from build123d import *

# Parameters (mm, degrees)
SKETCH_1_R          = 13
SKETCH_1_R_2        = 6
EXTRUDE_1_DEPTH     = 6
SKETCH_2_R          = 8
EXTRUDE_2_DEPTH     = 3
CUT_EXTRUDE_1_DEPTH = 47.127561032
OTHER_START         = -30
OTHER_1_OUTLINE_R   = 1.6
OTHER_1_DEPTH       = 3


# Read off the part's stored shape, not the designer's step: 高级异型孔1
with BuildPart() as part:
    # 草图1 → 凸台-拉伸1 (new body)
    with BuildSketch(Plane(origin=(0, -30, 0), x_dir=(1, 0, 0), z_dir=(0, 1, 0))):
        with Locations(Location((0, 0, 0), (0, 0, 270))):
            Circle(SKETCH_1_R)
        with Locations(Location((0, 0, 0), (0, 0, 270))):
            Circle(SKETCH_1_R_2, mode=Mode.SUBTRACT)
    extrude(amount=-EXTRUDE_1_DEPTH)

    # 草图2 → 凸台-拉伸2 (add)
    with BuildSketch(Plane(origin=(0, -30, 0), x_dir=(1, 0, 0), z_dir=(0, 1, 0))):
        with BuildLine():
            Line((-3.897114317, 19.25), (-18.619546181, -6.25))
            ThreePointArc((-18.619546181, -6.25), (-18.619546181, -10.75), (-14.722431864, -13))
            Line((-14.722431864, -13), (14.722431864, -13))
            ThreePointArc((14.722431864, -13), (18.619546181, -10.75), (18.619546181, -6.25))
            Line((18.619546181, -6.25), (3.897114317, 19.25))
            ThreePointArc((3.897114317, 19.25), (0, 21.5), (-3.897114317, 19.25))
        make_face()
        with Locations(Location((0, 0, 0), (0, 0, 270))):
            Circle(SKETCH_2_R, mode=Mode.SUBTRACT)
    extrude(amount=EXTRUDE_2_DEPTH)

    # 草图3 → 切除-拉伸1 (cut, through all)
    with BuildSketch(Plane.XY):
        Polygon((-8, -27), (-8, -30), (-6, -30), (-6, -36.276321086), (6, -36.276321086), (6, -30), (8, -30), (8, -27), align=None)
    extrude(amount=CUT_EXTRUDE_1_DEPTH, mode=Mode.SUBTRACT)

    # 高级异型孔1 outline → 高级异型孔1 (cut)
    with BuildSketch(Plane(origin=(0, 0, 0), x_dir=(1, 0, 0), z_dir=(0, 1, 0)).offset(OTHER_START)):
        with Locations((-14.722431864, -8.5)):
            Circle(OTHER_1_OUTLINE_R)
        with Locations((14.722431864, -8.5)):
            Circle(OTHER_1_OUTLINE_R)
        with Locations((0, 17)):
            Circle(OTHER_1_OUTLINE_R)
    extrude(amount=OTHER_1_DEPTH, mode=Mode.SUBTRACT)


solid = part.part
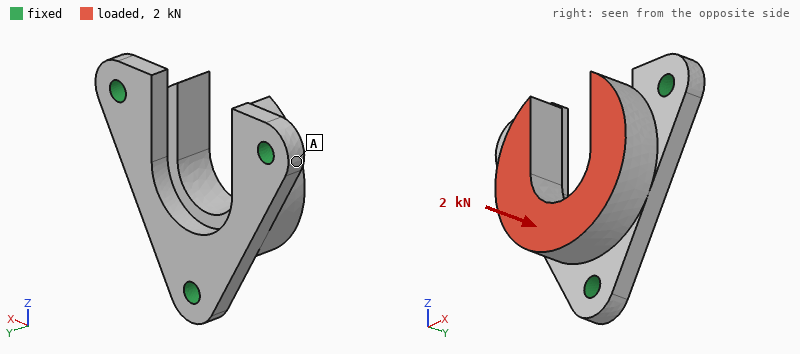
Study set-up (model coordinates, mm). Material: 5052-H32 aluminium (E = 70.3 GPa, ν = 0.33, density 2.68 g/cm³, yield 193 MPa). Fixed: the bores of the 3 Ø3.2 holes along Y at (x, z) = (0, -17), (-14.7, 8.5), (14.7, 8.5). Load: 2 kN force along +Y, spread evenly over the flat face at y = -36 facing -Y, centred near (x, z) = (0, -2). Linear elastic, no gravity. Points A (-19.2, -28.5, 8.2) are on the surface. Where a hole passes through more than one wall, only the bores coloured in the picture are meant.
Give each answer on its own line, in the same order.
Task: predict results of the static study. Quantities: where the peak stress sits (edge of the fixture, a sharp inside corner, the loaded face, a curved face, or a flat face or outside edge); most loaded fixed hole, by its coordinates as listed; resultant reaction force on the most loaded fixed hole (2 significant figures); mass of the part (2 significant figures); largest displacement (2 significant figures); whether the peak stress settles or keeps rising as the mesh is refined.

edge of the fixture
(0, -17)
1.0 kN
9.3 g
15 µm
keeps rising
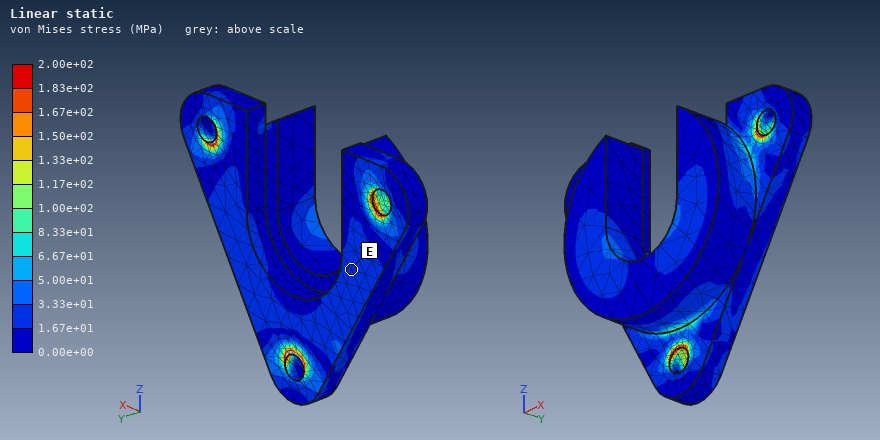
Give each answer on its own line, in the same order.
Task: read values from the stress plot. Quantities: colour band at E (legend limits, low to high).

1.67e+01 to 3.33e+01 MPa
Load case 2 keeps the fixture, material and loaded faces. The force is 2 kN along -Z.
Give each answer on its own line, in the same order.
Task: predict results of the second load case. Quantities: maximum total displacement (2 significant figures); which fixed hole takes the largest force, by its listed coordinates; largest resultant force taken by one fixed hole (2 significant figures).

20 µm
(0, -17)
1.1 kN
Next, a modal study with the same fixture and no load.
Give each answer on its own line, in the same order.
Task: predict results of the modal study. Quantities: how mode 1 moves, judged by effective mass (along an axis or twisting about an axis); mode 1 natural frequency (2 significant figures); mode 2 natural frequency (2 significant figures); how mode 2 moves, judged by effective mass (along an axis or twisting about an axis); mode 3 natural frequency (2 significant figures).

along X
17 kHz
22 kHz
along Y
25 kHz
